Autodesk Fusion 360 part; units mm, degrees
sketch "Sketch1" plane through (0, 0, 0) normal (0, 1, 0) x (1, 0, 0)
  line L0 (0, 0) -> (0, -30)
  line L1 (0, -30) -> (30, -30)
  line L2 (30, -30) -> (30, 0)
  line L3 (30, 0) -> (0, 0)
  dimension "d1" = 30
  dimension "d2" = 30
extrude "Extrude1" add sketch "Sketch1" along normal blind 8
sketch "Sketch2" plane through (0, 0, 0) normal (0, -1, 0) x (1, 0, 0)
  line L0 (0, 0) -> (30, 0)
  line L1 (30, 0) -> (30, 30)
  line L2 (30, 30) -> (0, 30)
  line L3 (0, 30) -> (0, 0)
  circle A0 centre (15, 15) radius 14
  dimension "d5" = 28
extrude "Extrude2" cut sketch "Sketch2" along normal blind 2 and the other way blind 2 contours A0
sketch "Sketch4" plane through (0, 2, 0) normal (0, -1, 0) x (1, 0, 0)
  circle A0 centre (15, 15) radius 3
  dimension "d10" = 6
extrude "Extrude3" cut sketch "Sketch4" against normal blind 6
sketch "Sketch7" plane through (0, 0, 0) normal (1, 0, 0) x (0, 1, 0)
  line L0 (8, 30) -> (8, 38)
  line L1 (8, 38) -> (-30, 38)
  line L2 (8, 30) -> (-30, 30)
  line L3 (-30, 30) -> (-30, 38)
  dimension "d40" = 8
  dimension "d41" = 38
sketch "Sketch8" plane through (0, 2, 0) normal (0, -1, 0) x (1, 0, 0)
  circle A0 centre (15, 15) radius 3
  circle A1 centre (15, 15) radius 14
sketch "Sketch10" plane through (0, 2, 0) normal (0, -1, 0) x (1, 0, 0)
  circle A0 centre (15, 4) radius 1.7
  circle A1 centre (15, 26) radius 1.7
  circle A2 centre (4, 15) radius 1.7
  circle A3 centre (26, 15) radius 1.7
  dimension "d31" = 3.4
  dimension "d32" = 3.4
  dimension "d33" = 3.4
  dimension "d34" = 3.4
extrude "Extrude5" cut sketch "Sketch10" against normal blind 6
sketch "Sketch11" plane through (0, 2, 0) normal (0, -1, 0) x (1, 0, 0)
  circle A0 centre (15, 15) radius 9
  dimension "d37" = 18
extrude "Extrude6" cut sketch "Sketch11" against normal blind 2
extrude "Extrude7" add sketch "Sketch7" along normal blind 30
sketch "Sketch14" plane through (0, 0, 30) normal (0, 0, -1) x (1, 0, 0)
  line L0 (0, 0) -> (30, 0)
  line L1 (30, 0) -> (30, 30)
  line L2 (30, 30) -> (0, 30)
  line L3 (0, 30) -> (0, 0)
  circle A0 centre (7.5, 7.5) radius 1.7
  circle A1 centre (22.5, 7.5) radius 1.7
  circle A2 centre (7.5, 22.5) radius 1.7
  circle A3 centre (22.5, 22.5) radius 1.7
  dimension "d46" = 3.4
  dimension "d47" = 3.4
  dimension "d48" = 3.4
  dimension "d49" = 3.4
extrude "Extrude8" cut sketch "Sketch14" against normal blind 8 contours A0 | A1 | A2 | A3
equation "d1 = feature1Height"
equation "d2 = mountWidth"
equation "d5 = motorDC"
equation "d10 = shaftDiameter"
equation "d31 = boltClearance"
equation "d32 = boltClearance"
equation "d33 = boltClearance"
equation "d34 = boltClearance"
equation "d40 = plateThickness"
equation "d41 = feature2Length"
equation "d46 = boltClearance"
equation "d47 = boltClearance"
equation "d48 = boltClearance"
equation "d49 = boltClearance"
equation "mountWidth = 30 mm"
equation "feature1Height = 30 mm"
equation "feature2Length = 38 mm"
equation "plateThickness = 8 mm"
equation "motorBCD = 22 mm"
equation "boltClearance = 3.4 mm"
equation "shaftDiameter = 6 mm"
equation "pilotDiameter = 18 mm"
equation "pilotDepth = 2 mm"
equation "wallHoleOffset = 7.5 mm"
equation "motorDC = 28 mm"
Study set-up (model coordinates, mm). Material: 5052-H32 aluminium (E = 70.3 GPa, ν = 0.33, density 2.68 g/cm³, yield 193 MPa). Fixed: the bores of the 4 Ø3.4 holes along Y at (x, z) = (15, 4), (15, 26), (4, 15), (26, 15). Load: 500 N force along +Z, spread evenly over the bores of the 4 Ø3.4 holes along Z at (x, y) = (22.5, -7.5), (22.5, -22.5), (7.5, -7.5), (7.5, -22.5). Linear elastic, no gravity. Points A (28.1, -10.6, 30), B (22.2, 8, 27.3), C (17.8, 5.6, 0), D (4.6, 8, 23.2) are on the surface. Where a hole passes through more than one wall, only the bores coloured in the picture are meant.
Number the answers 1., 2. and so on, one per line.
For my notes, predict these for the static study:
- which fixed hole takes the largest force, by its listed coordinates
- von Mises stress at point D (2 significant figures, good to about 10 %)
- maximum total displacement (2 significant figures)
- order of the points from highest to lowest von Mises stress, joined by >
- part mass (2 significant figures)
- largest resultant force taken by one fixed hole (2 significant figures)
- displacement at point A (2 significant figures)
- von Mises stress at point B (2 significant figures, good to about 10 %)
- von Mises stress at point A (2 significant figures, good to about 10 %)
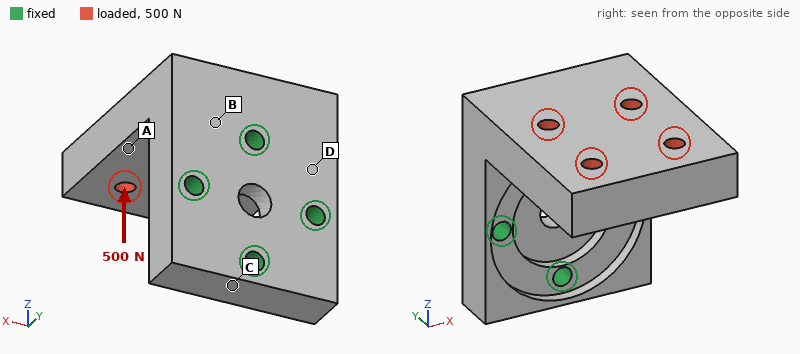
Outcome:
1. (15, 26)
2. 19 MPa
3. 80 µm
4. B > D > A > C
5. 37 g
6. 520 N
7. 29 µm
8. 26 MPa
9. 11 MPa
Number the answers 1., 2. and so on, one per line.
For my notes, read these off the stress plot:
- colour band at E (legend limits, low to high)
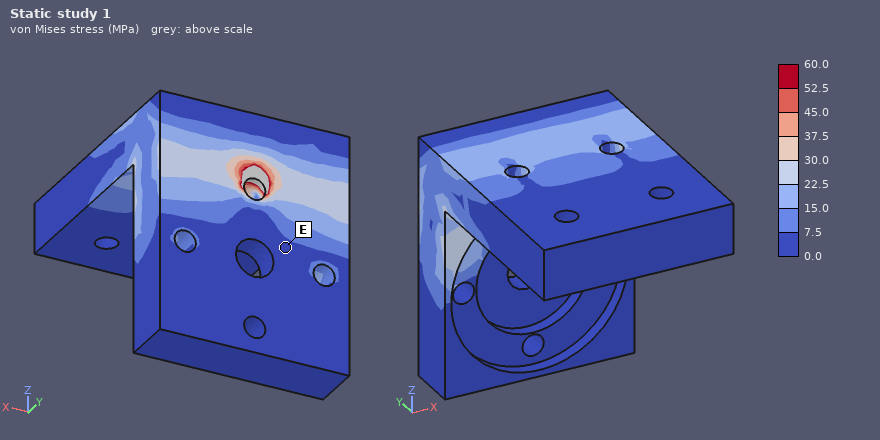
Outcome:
1. 0.0 to 7.5 MPa
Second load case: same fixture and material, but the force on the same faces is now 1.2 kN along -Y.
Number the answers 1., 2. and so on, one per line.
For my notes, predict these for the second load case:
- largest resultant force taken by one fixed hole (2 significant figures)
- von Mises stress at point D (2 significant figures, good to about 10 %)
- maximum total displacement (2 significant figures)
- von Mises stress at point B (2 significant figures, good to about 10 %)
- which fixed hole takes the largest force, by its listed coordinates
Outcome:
1. 1.4 kN
2. 17 MPa
3. 47 µm
4. 19 MPa
5. (15, 26)
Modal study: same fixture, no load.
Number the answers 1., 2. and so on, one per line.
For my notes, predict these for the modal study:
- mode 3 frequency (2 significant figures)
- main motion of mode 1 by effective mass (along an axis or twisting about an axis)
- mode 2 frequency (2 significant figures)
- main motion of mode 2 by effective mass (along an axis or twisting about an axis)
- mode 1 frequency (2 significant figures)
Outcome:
1. 12 kHz
2. along Z
3. 4800 Hz
4. along X
5. 3500 Hz
